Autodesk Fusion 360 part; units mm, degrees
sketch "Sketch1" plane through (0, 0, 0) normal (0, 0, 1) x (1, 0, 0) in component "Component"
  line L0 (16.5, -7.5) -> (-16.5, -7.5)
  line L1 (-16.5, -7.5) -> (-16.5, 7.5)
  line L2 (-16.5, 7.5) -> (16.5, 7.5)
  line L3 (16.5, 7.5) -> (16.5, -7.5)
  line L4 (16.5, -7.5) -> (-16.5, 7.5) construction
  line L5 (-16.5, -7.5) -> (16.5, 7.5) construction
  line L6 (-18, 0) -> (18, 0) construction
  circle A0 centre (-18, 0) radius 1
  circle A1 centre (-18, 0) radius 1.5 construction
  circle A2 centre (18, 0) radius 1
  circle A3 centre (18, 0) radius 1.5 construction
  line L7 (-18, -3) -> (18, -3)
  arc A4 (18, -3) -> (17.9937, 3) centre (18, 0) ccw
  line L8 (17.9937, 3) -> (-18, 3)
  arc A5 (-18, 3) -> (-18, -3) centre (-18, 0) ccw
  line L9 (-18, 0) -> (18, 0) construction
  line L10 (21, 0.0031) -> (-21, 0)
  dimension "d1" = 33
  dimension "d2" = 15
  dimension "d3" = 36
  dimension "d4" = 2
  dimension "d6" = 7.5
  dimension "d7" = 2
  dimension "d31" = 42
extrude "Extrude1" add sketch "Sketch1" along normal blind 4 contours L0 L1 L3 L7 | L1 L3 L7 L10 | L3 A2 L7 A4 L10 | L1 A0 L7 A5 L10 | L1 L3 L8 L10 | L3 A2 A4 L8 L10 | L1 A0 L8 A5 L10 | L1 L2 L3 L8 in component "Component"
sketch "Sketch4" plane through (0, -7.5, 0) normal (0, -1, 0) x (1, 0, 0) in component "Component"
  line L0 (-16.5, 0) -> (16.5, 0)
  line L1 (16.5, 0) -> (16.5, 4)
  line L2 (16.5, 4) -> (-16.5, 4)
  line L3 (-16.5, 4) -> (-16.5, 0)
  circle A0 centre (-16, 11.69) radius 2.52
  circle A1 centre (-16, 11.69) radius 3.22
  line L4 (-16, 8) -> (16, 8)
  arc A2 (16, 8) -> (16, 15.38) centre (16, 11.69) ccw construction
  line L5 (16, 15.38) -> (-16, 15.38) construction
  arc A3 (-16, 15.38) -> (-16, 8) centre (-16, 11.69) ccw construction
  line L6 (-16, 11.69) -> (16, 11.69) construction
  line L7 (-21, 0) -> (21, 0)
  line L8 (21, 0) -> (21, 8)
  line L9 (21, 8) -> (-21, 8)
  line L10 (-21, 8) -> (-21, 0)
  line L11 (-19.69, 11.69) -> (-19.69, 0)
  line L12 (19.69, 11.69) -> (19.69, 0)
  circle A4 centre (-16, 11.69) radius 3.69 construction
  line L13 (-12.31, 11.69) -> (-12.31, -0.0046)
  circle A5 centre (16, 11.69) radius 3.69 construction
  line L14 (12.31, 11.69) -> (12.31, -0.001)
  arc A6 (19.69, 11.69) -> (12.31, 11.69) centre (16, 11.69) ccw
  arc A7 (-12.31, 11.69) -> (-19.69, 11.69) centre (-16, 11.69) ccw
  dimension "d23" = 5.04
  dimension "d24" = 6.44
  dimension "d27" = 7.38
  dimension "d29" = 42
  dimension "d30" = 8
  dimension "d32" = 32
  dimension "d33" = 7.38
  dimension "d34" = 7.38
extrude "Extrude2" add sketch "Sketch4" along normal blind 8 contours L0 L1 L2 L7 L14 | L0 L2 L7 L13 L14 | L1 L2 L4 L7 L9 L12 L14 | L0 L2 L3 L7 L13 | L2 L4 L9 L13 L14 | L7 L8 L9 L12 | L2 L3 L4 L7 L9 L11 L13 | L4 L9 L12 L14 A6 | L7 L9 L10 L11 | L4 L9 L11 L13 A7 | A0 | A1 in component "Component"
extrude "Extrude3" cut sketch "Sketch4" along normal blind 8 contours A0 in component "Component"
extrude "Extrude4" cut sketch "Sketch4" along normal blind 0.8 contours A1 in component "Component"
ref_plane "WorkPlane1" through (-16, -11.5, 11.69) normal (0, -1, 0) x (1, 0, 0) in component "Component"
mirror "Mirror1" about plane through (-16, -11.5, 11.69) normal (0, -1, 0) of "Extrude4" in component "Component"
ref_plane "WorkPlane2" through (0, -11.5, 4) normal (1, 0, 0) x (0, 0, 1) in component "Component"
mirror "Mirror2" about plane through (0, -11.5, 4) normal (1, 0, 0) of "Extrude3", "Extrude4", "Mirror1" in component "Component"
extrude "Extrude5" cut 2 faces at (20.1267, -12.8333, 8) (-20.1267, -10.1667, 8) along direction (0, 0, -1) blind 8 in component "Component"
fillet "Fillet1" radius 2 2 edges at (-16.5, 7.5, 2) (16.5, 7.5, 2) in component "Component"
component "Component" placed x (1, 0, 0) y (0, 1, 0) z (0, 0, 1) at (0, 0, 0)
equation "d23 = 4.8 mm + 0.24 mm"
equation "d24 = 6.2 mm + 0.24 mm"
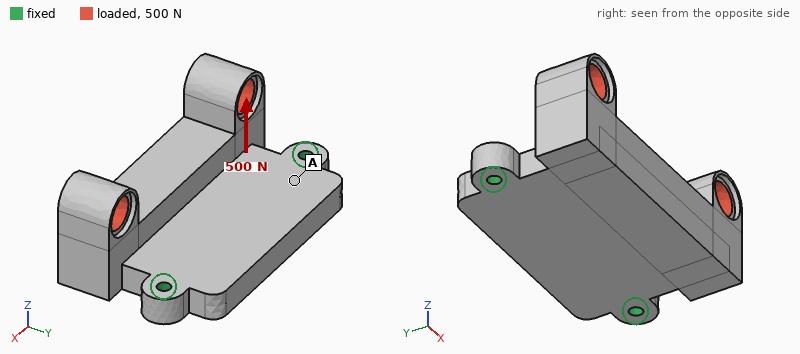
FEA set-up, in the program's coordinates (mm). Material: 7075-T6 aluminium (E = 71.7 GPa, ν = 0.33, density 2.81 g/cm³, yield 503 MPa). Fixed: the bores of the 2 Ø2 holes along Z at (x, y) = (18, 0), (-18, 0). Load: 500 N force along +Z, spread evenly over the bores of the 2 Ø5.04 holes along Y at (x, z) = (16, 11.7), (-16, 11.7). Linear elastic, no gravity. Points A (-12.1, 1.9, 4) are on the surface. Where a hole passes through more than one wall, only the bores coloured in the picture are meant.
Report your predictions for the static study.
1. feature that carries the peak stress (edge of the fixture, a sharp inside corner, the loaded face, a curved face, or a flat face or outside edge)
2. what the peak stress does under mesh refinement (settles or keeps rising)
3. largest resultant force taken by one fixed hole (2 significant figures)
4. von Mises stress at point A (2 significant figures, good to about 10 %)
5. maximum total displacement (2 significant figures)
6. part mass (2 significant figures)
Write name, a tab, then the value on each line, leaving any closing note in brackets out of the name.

feature that carries the peak stress	edge of the fixture
what the peak stress does under mesh refinement	keeps rising
largest resultant force taken by one fixed hole	250 N
von Mises stress at point A	37 MPa
maximum total displacement	0.13 mm
part mass	14 g
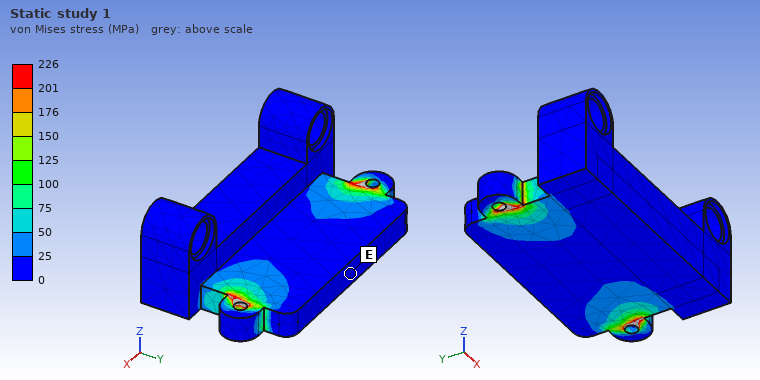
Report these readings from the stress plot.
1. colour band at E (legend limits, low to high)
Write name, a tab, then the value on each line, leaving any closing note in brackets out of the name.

colour band at E	0 to 25 MPa
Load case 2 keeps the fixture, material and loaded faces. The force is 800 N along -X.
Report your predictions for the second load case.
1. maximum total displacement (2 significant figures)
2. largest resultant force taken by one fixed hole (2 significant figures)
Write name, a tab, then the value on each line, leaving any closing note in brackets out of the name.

maximum total displacement	51 µm
largest resultant force taken by one fixed hole	540 N
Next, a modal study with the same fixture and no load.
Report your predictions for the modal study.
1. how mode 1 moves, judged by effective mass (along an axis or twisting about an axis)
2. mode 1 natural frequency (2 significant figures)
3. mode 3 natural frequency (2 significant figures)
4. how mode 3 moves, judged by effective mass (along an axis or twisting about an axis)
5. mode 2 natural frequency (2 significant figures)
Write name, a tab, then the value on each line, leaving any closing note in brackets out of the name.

how mode 1 moves, judged by effective mass	along Z
mode 1 natural frequency	4200 Hz
mode 3 natural frequency	13 kHz
how mode 3 moves, judged by effective mass	along Z
mode 2 natural frequency	9700 Hz
